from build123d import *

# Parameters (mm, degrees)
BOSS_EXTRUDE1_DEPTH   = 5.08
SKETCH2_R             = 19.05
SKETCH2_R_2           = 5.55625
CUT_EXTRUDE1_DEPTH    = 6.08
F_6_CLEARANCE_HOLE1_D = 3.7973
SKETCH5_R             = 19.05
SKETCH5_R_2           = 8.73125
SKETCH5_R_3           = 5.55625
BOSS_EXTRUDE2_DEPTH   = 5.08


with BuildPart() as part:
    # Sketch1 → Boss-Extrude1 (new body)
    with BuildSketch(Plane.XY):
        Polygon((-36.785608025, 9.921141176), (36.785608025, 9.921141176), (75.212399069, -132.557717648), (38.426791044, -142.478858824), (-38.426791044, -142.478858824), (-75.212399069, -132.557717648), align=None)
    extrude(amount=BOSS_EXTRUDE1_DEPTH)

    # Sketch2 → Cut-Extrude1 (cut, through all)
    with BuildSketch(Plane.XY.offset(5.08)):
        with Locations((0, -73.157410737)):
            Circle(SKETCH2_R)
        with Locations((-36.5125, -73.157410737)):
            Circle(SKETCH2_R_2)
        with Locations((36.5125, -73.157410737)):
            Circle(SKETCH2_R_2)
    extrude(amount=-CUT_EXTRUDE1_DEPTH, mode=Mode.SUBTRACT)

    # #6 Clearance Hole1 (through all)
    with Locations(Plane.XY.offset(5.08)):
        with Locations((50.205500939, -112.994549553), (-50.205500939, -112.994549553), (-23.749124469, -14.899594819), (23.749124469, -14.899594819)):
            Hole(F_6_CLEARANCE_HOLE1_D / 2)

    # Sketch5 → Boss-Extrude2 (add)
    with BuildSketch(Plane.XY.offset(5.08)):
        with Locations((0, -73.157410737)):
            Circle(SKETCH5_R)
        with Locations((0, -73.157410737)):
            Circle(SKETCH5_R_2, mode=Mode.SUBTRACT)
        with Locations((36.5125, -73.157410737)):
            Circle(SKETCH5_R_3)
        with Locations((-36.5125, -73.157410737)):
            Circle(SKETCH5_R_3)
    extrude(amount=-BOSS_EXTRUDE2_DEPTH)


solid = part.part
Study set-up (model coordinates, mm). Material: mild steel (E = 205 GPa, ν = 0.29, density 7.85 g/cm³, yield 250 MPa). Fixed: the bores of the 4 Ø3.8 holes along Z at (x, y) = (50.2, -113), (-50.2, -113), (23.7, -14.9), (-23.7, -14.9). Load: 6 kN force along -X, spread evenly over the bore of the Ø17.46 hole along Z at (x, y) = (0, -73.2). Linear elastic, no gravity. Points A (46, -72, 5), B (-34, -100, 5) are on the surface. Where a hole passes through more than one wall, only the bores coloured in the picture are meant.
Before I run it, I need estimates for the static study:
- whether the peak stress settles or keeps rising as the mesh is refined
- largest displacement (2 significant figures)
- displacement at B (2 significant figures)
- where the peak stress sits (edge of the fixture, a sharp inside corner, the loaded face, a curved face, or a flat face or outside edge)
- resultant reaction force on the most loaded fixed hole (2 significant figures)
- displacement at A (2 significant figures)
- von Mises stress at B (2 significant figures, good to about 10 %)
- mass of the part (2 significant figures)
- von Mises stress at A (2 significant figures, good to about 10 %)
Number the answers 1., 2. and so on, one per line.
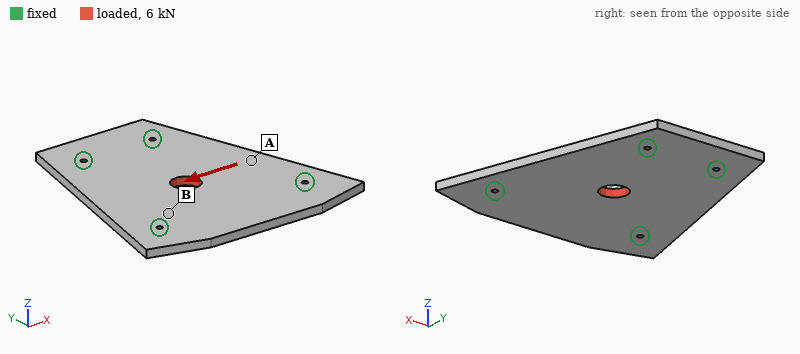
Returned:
1. keeps rising
2. 5.6 µm
3. 2.1 µm
4. edge of the fixture
5. 2.0 kN
6. 3.7 µm
7. 14 MPa
8. 670 g
9. 6.1 MPa
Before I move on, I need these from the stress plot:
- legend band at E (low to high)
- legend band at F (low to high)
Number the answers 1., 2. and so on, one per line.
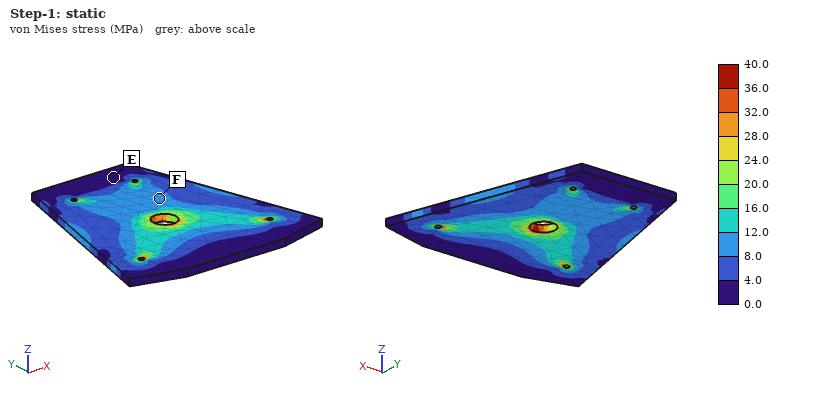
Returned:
1. 0.0 to 4.0 MPa
2. 8.0 to 12.0 MPa
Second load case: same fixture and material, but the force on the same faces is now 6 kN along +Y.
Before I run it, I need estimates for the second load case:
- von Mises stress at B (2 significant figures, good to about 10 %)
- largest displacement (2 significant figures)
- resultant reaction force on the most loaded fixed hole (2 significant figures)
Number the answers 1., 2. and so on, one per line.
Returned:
1. 8.6 MPa
2. 4.9 µm
3. 1.6 kN
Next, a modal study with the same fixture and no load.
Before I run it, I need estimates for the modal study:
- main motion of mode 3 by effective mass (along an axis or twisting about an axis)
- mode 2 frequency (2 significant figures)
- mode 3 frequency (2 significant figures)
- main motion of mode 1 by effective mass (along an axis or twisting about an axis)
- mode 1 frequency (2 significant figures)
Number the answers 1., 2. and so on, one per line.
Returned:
1. twisting about Y
2. 2100 Hz
3. 2600 Hz
4. along Z
5. 1900 Hz
